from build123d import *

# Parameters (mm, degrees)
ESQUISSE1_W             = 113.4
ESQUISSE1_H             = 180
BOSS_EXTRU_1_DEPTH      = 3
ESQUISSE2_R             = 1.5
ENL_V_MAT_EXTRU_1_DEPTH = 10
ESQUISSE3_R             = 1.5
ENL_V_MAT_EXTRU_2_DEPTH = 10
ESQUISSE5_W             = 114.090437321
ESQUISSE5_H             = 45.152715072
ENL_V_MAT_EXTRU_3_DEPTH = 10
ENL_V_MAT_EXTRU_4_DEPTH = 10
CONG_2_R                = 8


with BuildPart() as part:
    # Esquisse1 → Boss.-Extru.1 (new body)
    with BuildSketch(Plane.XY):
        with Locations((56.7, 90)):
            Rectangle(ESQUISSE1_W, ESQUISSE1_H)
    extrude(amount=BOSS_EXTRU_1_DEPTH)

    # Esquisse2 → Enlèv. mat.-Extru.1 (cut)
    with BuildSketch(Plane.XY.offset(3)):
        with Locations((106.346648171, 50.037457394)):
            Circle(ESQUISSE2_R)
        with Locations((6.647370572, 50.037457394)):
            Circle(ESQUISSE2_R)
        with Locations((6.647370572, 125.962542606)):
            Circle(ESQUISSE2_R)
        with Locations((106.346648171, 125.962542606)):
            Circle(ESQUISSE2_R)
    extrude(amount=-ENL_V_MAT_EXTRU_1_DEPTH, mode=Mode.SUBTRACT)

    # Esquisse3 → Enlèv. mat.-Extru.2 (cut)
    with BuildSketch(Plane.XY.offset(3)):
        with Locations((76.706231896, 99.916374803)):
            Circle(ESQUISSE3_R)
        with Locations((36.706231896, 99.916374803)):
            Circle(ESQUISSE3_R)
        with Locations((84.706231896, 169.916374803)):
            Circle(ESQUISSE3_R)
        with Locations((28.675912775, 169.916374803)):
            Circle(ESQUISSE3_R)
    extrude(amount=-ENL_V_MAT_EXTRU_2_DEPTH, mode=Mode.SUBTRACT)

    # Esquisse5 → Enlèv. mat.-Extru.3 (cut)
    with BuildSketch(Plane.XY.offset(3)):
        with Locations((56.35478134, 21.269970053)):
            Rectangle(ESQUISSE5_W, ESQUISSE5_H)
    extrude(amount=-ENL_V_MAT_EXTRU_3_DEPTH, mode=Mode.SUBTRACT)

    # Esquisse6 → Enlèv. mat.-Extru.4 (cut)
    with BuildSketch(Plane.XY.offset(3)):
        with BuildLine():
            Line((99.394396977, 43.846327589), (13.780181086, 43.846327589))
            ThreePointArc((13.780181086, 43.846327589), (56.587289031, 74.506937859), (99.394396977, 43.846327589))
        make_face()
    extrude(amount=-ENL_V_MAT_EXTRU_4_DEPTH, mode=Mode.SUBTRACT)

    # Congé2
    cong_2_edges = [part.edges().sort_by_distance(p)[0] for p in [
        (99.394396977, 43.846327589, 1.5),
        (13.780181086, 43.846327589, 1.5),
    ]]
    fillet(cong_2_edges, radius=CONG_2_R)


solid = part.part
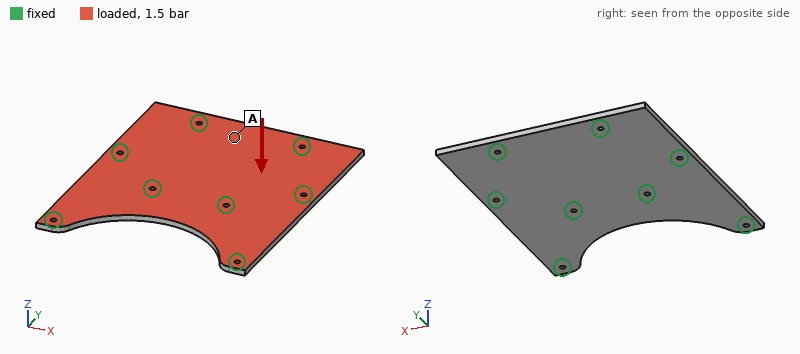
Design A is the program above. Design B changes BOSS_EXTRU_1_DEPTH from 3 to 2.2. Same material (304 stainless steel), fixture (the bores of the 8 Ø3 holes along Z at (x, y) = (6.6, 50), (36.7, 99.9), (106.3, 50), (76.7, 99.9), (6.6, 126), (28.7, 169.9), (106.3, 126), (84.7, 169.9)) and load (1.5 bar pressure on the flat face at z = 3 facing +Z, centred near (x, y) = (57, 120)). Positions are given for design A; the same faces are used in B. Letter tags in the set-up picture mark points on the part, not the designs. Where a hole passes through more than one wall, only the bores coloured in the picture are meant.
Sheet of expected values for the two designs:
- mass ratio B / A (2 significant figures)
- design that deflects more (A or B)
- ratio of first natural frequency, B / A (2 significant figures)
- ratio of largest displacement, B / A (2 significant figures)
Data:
0.73
B
0.75
2.5
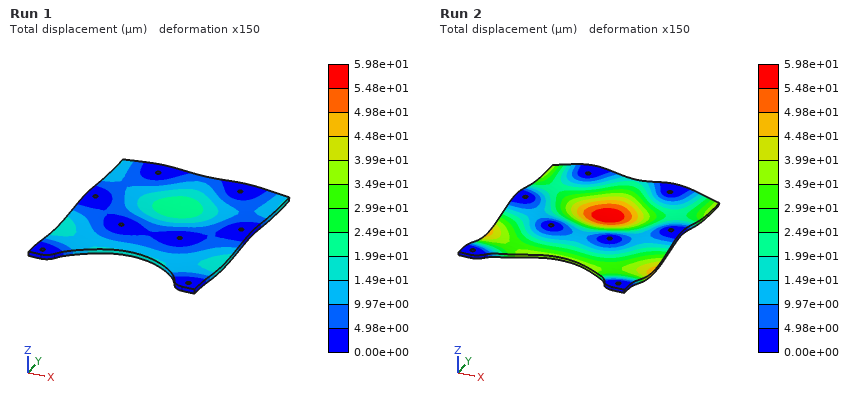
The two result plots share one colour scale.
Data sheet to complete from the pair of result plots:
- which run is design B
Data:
Run 2
